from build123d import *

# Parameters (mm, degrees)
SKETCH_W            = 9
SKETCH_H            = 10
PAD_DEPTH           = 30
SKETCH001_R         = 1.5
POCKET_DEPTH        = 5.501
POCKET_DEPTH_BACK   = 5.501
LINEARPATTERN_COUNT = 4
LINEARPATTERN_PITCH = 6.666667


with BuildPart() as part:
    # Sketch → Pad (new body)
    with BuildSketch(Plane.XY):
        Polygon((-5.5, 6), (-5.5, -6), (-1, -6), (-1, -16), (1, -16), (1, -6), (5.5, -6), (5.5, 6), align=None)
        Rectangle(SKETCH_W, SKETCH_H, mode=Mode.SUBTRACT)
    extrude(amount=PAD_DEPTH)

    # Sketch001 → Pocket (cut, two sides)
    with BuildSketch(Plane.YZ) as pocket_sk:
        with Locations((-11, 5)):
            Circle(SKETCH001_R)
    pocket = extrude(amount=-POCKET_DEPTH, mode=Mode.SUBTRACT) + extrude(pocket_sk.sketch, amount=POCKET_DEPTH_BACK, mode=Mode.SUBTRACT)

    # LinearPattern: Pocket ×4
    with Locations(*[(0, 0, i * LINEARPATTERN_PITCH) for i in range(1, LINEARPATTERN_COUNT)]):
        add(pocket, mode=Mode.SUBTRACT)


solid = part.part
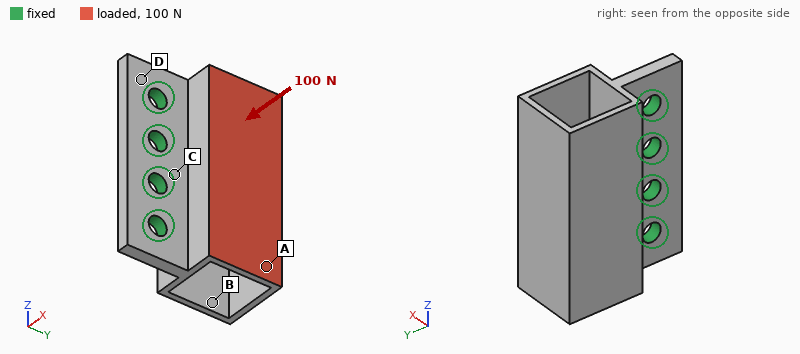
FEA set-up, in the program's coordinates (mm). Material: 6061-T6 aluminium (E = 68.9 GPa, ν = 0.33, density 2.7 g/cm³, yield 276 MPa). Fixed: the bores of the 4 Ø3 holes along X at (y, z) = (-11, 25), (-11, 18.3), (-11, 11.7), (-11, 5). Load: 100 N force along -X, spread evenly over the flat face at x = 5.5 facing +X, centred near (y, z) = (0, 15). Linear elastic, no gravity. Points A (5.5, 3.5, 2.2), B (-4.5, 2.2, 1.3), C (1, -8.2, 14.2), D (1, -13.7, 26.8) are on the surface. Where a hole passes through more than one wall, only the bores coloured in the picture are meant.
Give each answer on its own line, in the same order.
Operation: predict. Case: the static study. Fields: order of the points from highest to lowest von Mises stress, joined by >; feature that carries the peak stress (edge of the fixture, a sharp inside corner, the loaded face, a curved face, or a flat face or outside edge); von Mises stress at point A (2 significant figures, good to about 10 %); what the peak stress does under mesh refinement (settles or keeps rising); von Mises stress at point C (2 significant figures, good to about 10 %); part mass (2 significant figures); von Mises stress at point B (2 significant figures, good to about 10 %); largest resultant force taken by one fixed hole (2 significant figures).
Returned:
C > A > B > D
edge of the fixture
20 MPa
keeps rising
34 MPa
4.9 g
12 MPa
26 N
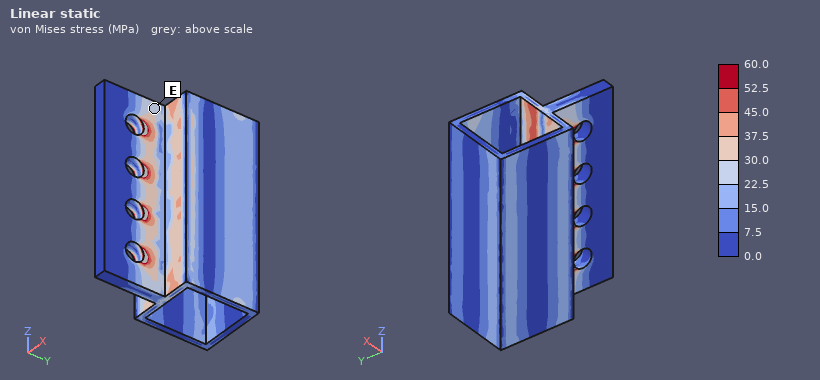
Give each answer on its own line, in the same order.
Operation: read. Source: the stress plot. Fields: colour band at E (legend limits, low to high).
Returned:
22.5 to 30.0 MPa
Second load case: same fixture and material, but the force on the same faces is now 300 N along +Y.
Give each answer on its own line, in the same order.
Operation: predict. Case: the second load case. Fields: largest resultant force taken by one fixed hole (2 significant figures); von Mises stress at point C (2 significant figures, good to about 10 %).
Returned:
88 N
72 MPa
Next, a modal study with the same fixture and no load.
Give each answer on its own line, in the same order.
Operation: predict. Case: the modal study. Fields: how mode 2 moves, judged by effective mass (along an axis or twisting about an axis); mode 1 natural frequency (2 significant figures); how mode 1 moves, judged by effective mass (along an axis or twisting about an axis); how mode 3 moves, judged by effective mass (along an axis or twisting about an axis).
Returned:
along Z
3000 Hz
along X
twisting about Y
